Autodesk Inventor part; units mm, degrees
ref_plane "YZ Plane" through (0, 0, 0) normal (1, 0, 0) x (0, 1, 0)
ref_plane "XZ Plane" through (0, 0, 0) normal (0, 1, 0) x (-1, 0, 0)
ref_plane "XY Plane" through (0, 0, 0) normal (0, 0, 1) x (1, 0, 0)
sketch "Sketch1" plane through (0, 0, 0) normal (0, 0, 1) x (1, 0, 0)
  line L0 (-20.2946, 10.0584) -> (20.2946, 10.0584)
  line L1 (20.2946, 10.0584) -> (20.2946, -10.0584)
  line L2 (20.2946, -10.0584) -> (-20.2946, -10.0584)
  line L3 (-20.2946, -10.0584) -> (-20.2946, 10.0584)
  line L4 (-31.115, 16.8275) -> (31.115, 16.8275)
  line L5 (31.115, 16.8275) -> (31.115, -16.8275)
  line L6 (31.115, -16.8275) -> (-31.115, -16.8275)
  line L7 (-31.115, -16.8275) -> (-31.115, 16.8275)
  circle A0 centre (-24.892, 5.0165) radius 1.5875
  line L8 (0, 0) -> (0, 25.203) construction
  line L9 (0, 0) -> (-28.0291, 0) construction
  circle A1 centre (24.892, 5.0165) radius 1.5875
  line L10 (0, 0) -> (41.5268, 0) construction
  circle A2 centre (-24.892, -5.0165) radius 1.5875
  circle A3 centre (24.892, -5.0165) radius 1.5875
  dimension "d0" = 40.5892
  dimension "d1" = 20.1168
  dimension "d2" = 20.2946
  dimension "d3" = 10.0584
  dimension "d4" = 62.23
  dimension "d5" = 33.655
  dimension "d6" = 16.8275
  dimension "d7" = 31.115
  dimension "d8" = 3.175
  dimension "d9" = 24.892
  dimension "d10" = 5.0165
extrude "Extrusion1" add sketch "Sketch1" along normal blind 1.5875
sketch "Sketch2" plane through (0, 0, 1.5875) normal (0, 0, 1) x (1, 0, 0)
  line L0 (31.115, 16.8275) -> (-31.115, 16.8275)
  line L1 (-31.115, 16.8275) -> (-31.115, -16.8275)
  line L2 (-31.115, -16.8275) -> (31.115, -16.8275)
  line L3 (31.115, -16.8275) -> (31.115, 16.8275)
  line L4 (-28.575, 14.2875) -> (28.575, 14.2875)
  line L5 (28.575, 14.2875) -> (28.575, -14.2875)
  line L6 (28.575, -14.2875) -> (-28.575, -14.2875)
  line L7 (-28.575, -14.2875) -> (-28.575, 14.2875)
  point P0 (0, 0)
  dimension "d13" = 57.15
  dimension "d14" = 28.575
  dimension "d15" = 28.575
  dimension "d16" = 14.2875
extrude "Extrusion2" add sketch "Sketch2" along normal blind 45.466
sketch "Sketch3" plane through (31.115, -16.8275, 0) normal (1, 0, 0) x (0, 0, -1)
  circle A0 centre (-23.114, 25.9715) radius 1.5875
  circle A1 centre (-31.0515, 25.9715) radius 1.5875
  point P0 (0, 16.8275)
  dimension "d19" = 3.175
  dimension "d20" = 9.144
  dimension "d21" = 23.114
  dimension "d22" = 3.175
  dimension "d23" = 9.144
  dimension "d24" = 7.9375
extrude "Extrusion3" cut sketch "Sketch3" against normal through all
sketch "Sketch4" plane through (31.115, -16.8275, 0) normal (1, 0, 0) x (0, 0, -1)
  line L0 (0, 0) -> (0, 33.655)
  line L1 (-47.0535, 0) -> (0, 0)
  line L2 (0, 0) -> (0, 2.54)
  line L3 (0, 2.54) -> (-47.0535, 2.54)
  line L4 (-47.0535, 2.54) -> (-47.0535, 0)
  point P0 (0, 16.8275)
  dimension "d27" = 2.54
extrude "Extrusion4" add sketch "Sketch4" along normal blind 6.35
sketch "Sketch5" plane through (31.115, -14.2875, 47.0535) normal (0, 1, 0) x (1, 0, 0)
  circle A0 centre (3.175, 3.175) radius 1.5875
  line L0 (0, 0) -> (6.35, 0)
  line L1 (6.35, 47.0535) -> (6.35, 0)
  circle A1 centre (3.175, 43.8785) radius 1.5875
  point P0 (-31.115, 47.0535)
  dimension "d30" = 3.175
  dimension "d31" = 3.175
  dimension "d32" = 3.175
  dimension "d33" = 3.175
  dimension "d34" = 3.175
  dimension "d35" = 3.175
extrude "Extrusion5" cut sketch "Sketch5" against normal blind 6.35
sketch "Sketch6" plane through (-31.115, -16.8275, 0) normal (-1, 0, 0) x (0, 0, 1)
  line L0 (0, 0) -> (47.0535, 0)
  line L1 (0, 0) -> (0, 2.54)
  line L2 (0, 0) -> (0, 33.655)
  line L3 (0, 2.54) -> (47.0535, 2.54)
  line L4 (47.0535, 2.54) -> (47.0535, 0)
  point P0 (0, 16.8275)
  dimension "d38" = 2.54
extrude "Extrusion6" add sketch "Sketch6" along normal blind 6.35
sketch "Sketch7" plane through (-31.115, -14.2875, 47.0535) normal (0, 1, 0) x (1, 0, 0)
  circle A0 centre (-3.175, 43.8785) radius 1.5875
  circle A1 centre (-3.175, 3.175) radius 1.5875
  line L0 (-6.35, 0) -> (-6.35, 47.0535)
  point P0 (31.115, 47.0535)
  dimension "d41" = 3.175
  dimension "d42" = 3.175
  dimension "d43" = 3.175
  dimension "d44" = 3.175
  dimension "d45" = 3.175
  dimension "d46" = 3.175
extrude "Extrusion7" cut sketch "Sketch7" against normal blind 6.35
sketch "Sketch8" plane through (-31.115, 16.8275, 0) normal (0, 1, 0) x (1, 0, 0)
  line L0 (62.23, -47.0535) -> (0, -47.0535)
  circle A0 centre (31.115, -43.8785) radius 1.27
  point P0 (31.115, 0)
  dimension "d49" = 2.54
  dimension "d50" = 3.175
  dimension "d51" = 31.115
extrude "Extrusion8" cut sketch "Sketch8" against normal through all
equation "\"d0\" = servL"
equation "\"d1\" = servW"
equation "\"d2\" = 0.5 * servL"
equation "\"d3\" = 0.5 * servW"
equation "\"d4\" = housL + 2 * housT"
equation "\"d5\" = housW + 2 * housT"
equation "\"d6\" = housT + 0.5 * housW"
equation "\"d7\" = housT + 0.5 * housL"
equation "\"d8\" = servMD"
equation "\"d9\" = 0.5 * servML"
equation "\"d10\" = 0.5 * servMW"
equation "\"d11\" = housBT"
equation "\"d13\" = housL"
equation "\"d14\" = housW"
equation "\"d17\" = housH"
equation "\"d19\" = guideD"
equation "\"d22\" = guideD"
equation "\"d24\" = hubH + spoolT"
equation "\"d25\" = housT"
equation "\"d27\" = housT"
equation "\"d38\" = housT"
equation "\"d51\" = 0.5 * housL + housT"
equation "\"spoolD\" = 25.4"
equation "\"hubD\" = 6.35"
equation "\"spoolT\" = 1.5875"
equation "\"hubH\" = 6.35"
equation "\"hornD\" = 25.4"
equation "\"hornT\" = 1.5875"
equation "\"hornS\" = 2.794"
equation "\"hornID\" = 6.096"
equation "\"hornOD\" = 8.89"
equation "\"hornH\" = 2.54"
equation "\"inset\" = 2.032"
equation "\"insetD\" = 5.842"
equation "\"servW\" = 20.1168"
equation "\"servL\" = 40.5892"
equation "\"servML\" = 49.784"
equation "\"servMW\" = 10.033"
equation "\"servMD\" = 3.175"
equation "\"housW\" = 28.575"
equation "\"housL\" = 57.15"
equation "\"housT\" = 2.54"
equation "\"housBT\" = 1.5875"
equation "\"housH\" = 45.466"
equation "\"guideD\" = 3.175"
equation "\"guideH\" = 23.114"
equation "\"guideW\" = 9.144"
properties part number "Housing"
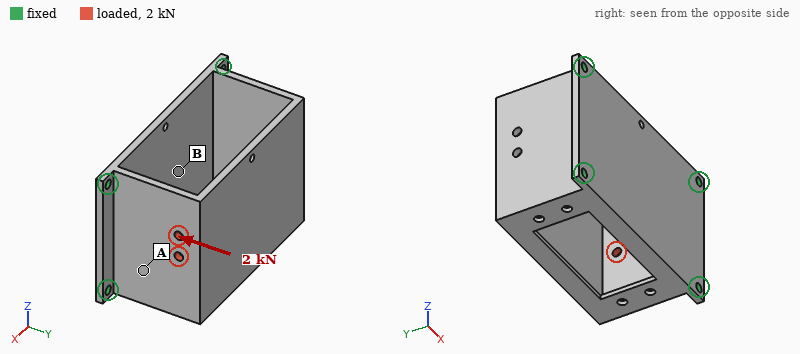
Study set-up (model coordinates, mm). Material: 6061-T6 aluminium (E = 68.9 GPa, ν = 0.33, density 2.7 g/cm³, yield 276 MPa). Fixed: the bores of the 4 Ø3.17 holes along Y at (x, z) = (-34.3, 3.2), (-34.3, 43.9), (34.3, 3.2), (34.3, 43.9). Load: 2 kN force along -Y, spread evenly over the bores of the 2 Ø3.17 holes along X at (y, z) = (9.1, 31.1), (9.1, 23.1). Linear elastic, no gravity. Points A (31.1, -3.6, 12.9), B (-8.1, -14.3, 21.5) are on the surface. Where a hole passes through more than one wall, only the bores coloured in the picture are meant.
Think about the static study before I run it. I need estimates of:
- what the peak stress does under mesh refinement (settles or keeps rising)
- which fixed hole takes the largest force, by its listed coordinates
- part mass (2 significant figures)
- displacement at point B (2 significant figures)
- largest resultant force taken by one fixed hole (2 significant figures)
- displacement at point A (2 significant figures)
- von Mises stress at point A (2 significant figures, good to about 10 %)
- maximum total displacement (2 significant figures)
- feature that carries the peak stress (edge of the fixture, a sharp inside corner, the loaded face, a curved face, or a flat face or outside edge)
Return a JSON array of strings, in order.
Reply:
["keeps rising", "(34.3, 43.9)", "66 g", "18 µm", "1.2 kN", "23 µm", "24 MPa", "56 µm", "edge of the fixture"]
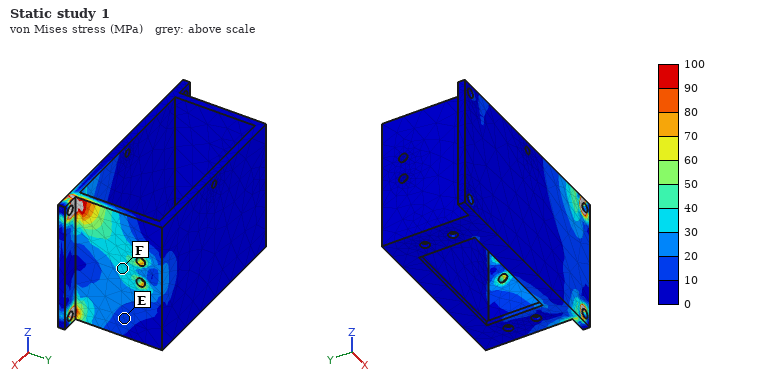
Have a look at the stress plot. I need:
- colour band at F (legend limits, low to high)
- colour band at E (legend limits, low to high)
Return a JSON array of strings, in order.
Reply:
["30 to 40 MPa", "10 to 20 MPa"]
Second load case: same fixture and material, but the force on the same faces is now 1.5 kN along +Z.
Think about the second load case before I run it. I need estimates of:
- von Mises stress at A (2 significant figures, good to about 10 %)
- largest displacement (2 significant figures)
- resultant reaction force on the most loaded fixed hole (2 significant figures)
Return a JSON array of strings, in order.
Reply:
["30 MPa", "64 µm", "1.2 kN"]
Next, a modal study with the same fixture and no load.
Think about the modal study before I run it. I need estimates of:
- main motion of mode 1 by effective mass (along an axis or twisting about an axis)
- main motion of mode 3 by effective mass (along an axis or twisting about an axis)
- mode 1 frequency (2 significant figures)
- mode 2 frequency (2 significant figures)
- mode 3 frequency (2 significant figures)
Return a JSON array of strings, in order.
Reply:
["along X", "along Y", "2200 Hz", "3100 Hz", "3300 Hz"]
